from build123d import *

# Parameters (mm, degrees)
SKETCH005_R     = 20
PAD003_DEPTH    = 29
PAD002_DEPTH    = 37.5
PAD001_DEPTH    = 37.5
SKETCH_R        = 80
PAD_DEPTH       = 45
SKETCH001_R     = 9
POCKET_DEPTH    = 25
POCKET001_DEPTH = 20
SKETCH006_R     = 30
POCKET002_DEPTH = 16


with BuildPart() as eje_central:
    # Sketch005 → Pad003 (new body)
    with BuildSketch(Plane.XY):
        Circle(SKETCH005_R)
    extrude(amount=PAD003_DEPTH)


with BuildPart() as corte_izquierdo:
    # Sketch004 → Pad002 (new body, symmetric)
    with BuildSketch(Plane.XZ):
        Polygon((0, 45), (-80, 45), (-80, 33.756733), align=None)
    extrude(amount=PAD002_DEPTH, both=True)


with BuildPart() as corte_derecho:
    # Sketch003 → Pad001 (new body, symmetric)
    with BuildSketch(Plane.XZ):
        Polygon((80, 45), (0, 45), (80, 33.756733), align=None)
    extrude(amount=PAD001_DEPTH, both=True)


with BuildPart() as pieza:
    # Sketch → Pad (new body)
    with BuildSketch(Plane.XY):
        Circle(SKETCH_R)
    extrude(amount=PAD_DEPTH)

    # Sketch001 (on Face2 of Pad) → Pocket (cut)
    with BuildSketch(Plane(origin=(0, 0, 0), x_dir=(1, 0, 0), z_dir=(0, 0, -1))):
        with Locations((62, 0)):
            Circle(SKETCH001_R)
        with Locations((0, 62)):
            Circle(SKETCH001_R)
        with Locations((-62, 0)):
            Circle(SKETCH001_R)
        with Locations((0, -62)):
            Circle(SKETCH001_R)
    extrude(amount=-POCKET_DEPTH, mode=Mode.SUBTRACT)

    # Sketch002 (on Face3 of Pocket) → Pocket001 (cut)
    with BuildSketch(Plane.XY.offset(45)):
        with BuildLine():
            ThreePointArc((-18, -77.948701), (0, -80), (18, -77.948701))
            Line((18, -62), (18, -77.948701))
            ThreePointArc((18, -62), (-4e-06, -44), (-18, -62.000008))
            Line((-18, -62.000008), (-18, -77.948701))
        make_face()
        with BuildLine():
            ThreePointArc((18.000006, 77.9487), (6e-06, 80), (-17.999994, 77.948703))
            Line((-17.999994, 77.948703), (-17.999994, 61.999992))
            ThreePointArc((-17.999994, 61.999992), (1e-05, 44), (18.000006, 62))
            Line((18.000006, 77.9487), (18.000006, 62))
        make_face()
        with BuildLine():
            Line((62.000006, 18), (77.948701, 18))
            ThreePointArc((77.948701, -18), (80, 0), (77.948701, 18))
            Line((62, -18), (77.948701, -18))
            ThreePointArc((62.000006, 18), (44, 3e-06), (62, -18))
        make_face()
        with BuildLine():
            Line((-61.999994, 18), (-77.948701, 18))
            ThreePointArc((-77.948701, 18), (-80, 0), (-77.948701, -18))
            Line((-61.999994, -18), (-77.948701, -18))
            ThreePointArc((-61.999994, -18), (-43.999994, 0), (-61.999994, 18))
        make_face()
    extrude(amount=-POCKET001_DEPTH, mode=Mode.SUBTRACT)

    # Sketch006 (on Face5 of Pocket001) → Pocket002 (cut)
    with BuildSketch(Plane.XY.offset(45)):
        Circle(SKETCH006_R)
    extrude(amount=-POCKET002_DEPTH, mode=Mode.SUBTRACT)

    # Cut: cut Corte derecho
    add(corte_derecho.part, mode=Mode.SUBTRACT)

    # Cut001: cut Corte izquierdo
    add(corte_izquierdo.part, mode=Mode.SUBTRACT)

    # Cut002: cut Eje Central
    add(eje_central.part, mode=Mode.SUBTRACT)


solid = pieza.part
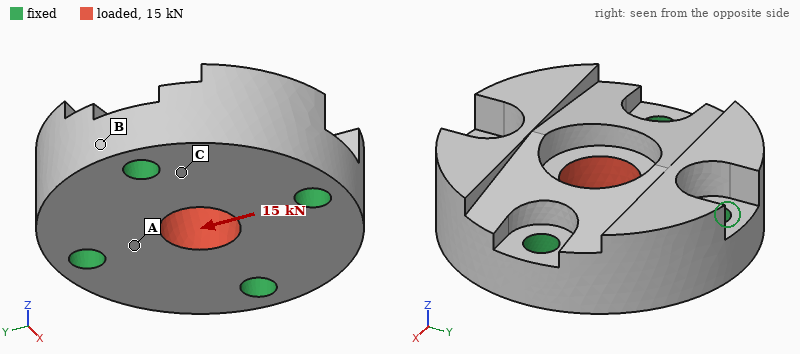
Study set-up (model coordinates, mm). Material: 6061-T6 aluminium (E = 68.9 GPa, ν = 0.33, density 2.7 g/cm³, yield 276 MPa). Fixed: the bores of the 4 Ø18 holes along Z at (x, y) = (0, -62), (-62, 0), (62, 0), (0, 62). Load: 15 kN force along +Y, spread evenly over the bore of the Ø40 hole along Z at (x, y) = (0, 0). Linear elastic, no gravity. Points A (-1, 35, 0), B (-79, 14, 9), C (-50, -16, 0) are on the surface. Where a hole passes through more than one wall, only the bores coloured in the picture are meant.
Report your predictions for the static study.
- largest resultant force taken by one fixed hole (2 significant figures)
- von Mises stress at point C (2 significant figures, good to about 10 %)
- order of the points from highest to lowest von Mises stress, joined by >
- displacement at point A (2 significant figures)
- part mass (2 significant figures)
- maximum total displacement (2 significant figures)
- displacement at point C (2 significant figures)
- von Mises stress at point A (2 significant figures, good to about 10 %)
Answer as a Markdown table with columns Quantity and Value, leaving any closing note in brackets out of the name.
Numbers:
| Quantity | Value |
|---|---|
| largest resultant force taken by one fixed hole | 4.8 kN |
| von Mises stress at point C | 1.8 MPa |
| order of the points from highest to lowest von Mises stress, joined by > | A > C > B |
| displacement at point A | 1.5 µm |
| part mass | 1.8 kg |
| maximum total displacement | 3.0 µm |
| displacement at point C | 0.69 µm |
| von Mises stress at point A | 5.3 MPa |
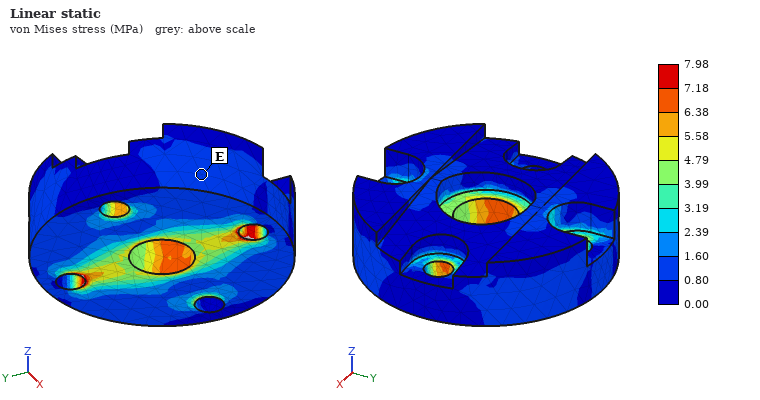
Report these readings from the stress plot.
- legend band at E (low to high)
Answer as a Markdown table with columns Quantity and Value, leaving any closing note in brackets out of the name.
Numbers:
| Quantity | Value |
|---|---|
| legend band at E | 0.80 to 1.60 MPa |
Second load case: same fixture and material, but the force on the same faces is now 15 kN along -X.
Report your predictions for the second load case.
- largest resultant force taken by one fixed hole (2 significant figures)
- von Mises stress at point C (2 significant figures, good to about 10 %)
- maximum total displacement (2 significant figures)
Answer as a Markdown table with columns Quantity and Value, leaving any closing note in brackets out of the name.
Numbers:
| Quantity | Value |
|---|---|
| largest resultant force taken by one fixed hole | 4.8 kN |
| von Mises stress at point C | 2.3 MPa |
| maximum total displacement | 3.0 µm |
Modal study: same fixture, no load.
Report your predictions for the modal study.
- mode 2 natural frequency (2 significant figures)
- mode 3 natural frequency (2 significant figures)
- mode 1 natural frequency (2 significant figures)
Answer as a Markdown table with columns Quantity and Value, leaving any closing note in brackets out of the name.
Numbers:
| Quantity | Value |
|---|---|
| mode 2 natural frequency | 9400 Hz |
| mode 3 natural frequency | 9600 Hz |
| mode 1 natural frequency | 8800 Hz |
